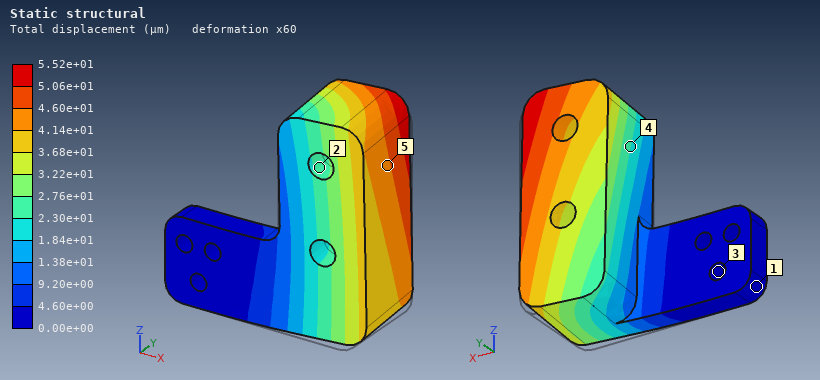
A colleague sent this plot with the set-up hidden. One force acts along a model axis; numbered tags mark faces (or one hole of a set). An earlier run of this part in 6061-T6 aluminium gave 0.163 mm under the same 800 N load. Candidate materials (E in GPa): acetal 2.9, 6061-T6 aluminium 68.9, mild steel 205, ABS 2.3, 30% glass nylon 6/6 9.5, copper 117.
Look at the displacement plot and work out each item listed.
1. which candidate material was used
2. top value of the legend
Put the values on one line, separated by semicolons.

mild steel; 5.52e+01 µm
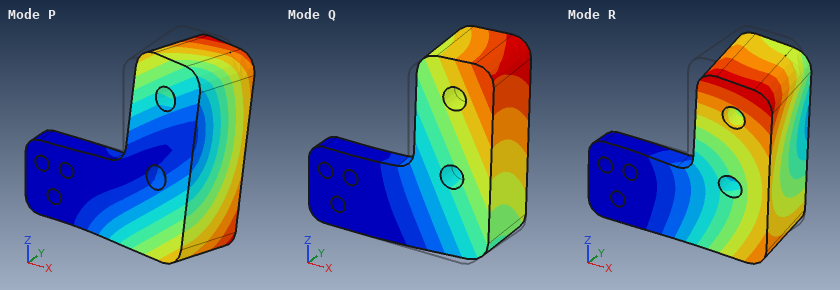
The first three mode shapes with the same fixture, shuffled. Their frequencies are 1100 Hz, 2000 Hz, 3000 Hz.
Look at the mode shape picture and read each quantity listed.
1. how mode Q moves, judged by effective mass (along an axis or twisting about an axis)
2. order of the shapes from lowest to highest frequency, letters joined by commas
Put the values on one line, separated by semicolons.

along Y; Q, P, R
